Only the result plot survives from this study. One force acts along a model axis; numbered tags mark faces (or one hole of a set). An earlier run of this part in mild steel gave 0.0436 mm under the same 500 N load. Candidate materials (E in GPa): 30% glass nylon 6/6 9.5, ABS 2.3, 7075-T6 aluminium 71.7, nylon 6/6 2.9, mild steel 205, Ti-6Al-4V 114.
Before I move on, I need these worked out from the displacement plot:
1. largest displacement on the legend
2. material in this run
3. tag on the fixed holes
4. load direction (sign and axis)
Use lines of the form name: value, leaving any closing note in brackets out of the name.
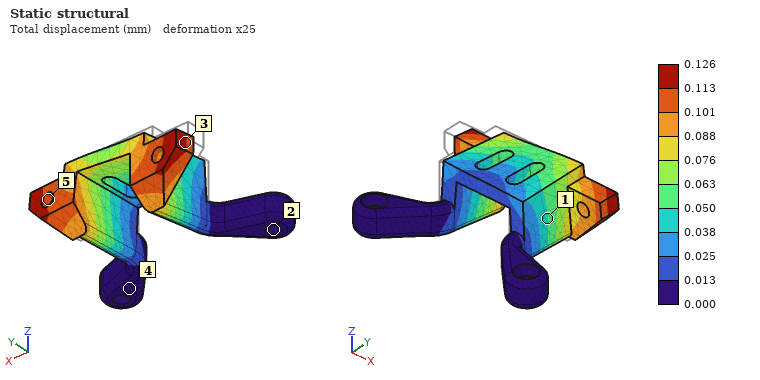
largest displacement on the legend: 0.126 mm
material in this run: 7075-T6 aluminium
tag on the fixed holes: 2
load direction: +X
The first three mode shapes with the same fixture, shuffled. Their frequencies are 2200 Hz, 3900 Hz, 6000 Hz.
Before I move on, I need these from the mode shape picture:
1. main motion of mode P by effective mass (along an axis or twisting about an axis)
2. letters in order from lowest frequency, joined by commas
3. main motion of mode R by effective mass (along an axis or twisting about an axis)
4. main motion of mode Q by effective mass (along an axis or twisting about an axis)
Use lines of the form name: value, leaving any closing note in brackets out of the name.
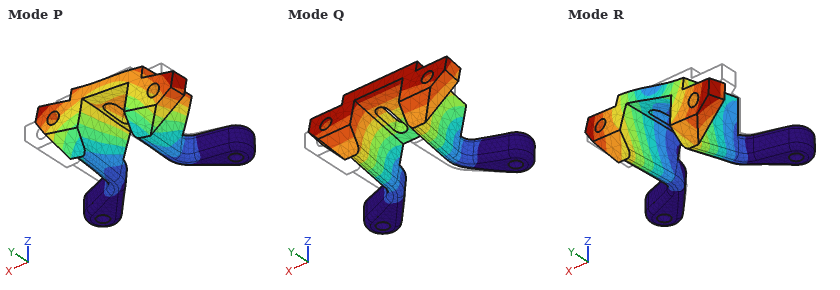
main motion of mode P by effective mass: along X
letters in order from lowest frequency, joined by commas: Q, R, P
main motion of mode R by effective mass: along X
main motion of mode Q by effective mass: along Z
